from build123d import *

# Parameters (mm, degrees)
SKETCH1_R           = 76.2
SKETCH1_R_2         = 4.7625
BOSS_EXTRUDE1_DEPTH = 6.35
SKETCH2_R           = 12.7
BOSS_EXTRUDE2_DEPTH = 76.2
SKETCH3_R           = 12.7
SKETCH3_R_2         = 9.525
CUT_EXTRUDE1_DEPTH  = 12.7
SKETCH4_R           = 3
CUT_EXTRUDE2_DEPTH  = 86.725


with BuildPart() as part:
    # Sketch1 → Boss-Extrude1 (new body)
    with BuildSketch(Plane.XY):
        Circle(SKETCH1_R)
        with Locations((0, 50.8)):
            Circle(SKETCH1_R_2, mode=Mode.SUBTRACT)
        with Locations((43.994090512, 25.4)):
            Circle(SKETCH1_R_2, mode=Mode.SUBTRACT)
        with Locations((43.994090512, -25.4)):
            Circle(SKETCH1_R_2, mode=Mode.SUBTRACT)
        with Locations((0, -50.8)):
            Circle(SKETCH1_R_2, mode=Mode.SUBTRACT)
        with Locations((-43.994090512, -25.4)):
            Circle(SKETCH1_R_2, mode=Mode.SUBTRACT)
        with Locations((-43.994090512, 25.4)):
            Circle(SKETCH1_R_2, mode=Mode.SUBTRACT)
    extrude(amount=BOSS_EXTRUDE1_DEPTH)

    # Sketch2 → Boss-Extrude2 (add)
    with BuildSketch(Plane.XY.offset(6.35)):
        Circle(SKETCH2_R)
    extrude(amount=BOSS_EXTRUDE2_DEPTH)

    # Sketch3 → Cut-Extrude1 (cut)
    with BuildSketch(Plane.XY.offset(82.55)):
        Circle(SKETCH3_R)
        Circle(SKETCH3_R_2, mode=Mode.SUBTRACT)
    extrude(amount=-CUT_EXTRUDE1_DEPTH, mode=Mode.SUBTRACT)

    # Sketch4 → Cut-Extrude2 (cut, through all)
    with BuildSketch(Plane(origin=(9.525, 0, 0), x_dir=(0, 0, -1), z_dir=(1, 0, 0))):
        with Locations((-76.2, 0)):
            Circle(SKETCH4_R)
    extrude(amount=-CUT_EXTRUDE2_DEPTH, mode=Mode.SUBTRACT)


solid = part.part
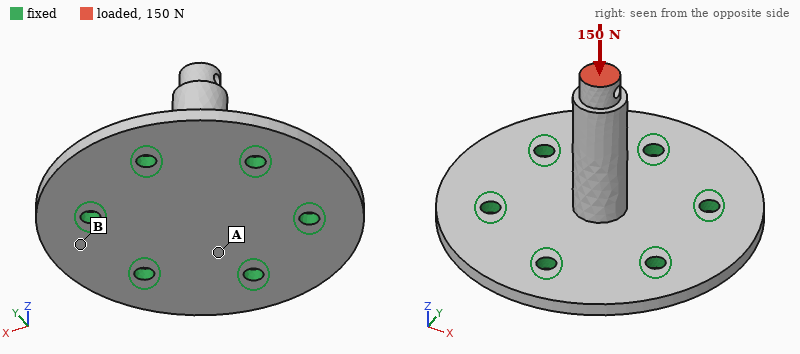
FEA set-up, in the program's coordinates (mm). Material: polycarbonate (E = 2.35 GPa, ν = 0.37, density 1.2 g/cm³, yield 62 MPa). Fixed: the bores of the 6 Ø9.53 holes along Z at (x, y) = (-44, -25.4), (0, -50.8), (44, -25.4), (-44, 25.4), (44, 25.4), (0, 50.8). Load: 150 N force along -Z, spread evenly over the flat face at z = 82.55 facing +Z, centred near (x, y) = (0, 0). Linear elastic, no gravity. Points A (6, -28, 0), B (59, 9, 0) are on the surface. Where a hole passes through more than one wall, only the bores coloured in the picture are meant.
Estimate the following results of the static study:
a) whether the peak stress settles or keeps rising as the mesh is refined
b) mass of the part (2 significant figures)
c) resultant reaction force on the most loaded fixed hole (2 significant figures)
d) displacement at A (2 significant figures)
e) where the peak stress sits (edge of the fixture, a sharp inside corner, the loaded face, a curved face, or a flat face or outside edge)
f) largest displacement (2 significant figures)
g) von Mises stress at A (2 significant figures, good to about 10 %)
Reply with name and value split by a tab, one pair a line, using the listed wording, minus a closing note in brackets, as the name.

whether the peak stress settles or keeps rising as the mesh is refined	keeps rising
mass of the part	180 g
resultant reaction force on the most loaded fixed hole	26 N
displacement at A	39 µm
where the peak stress sits	edge of the fixture
largest displacement	93 µm
von Mises stress at A	0.68 MPa
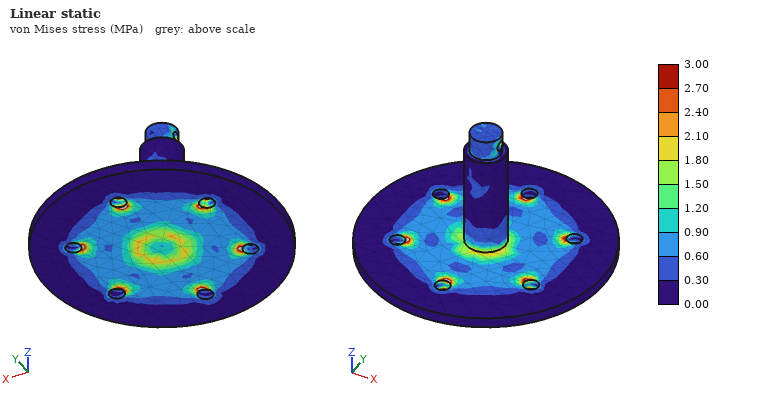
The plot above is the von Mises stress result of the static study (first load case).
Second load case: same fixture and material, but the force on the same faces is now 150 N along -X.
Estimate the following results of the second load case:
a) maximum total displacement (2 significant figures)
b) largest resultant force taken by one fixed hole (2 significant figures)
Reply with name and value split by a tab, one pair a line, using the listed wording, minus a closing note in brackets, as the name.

maximum total displacement	1.5 mm
largest resultant force taken by one fixed hole	100 N
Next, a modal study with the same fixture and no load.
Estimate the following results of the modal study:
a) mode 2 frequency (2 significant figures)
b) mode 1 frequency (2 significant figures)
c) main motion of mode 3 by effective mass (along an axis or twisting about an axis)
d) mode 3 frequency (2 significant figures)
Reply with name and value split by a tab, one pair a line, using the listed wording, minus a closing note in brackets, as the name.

mode 2 frequency	480 Hz
mode 1 frequency	470 Hz
main motion of mode 3 by effective mass	along Z
mode 3 frequency	910 Hz
